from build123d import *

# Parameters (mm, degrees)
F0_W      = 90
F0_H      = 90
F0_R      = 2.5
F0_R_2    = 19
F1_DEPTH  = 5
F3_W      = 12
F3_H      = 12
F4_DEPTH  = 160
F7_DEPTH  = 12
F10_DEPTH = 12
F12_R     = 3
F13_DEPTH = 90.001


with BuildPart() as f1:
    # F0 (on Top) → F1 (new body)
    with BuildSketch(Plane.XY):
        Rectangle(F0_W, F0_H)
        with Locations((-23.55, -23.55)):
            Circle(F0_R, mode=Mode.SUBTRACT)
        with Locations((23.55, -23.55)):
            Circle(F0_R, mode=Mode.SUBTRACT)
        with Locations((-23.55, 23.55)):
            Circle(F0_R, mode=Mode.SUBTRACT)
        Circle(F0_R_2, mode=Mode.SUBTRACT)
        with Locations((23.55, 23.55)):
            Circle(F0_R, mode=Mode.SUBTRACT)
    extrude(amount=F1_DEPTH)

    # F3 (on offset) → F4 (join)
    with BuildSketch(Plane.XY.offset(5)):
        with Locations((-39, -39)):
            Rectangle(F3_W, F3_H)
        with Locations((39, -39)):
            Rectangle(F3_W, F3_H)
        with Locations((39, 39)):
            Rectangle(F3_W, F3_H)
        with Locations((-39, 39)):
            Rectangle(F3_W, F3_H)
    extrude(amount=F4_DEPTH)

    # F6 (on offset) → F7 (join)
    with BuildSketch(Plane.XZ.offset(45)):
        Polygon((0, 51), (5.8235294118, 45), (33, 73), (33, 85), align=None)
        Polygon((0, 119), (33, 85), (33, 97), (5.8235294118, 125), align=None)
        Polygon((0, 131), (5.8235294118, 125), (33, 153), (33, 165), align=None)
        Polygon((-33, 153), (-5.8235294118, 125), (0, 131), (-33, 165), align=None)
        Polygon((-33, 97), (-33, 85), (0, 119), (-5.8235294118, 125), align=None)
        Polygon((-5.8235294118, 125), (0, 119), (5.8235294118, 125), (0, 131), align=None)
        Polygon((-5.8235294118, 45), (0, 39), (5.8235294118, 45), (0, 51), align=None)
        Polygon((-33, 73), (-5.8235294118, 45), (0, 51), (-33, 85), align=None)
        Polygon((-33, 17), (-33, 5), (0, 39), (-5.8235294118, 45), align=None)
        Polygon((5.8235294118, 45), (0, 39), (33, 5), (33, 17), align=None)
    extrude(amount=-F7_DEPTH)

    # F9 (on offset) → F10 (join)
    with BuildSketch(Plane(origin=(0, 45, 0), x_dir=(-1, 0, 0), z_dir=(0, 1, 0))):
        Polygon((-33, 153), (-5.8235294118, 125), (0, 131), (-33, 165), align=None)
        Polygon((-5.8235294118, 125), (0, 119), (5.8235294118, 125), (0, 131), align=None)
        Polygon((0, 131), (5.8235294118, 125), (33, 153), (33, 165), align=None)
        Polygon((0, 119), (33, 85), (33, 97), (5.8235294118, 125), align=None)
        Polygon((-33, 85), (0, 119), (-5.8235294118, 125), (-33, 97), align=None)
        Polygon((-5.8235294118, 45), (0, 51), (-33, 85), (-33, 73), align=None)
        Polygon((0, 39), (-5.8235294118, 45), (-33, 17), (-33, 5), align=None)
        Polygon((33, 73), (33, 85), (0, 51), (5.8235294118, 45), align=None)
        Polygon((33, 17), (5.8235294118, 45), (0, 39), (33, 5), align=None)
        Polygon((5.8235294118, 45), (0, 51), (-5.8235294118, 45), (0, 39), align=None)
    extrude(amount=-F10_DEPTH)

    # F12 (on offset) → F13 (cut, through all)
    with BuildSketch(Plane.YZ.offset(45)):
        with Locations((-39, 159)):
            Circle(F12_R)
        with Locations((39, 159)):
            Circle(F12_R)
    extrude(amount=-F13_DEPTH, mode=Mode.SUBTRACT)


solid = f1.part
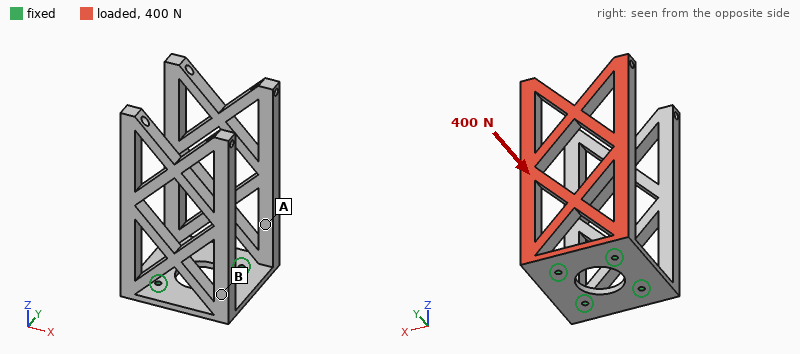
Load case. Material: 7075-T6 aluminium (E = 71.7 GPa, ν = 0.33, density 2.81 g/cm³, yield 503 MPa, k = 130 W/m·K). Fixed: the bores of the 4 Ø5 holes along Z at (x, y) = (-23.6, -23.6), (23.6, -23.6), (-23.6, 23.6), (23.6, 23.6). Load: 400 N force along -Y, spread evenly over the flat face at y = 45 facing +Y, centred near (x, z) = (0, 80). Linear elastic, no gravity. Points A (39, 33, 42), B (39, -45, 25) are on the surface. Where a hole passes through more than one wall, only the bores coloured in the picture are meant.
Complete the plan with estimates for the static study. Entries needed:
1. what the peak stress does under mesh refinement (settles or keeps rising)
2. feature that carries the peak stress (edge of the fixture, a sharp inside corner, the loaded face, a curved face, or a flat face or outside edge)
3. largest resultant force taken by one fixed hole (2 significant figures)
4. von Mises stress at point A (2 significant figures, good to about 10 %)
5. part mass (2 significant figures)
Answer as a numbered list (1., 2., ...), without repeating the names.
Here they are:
1. keeps rising
2. edge of the fixture
3. 190 N
4. 23 MPa
5. 550 g
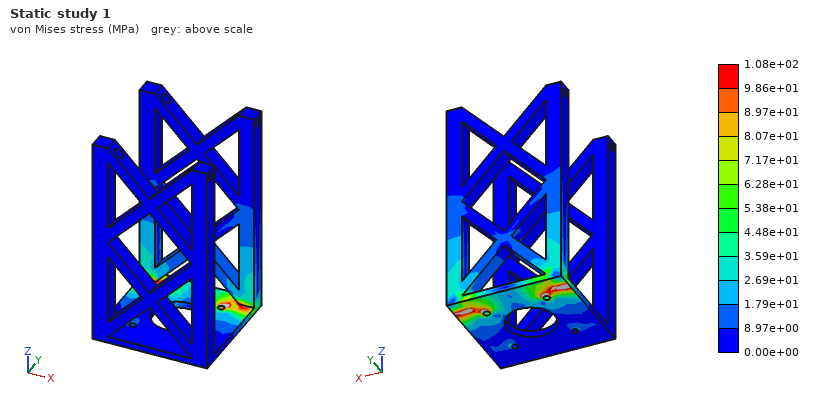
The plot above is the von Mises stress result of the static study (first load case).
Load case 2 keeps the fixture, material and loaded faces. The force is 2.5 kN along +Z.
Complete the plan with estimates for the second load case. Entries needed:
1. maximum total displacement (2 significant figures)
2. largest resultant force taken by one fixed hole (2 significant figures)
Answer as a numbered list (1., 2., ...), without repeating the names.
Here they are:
1. 2.3 mm
2. 1.4 kN
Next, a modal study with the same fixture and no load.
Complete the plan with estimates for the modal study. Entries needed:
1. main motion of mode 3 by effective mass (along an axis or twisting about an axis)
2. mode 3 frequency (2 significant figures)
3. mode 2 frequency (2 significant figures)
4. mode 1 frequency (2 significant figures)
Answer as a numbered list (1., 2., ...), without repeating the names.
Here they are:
1. along X
2. 620 Hz
3. 170 Hz
4. 170 Hz
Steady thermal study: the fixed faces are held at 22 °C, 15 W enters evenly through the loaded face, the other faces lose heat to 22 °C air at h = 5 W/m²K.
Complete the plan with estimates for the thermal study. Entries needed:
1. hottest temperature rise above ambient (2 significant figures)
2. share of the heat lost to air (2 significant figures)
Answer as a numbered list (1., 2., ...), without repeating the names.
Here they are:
1. 25 K
2. 15 %
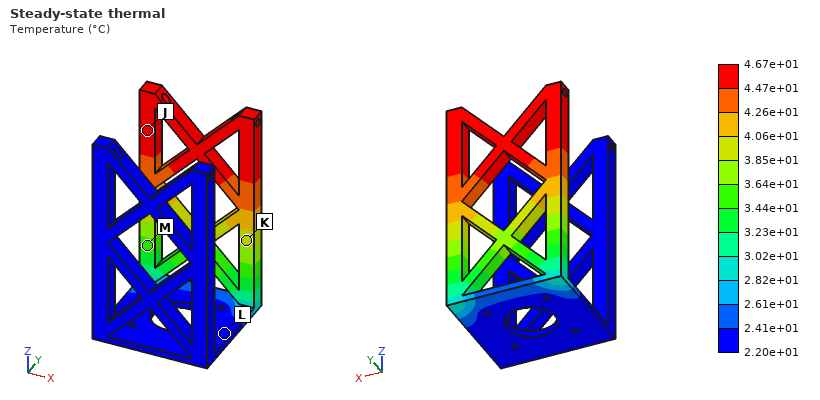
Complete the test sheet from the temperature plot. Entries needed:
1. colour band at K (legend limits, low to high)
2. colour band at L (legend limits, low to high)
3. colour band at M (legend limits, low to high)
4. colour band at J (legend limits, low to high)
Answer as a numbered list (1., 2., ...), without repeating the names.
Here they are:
1. 3.85e+01 to 4.06e+01 °C
2. 2.20e+01 to 2.41e+01 °C
3. 3.44e+01 to 3.64e+01 °C
4. 4.47e+01 to 4.67e+01 °C
